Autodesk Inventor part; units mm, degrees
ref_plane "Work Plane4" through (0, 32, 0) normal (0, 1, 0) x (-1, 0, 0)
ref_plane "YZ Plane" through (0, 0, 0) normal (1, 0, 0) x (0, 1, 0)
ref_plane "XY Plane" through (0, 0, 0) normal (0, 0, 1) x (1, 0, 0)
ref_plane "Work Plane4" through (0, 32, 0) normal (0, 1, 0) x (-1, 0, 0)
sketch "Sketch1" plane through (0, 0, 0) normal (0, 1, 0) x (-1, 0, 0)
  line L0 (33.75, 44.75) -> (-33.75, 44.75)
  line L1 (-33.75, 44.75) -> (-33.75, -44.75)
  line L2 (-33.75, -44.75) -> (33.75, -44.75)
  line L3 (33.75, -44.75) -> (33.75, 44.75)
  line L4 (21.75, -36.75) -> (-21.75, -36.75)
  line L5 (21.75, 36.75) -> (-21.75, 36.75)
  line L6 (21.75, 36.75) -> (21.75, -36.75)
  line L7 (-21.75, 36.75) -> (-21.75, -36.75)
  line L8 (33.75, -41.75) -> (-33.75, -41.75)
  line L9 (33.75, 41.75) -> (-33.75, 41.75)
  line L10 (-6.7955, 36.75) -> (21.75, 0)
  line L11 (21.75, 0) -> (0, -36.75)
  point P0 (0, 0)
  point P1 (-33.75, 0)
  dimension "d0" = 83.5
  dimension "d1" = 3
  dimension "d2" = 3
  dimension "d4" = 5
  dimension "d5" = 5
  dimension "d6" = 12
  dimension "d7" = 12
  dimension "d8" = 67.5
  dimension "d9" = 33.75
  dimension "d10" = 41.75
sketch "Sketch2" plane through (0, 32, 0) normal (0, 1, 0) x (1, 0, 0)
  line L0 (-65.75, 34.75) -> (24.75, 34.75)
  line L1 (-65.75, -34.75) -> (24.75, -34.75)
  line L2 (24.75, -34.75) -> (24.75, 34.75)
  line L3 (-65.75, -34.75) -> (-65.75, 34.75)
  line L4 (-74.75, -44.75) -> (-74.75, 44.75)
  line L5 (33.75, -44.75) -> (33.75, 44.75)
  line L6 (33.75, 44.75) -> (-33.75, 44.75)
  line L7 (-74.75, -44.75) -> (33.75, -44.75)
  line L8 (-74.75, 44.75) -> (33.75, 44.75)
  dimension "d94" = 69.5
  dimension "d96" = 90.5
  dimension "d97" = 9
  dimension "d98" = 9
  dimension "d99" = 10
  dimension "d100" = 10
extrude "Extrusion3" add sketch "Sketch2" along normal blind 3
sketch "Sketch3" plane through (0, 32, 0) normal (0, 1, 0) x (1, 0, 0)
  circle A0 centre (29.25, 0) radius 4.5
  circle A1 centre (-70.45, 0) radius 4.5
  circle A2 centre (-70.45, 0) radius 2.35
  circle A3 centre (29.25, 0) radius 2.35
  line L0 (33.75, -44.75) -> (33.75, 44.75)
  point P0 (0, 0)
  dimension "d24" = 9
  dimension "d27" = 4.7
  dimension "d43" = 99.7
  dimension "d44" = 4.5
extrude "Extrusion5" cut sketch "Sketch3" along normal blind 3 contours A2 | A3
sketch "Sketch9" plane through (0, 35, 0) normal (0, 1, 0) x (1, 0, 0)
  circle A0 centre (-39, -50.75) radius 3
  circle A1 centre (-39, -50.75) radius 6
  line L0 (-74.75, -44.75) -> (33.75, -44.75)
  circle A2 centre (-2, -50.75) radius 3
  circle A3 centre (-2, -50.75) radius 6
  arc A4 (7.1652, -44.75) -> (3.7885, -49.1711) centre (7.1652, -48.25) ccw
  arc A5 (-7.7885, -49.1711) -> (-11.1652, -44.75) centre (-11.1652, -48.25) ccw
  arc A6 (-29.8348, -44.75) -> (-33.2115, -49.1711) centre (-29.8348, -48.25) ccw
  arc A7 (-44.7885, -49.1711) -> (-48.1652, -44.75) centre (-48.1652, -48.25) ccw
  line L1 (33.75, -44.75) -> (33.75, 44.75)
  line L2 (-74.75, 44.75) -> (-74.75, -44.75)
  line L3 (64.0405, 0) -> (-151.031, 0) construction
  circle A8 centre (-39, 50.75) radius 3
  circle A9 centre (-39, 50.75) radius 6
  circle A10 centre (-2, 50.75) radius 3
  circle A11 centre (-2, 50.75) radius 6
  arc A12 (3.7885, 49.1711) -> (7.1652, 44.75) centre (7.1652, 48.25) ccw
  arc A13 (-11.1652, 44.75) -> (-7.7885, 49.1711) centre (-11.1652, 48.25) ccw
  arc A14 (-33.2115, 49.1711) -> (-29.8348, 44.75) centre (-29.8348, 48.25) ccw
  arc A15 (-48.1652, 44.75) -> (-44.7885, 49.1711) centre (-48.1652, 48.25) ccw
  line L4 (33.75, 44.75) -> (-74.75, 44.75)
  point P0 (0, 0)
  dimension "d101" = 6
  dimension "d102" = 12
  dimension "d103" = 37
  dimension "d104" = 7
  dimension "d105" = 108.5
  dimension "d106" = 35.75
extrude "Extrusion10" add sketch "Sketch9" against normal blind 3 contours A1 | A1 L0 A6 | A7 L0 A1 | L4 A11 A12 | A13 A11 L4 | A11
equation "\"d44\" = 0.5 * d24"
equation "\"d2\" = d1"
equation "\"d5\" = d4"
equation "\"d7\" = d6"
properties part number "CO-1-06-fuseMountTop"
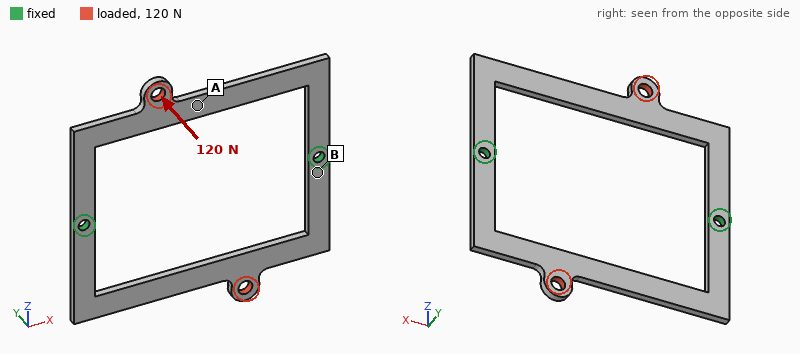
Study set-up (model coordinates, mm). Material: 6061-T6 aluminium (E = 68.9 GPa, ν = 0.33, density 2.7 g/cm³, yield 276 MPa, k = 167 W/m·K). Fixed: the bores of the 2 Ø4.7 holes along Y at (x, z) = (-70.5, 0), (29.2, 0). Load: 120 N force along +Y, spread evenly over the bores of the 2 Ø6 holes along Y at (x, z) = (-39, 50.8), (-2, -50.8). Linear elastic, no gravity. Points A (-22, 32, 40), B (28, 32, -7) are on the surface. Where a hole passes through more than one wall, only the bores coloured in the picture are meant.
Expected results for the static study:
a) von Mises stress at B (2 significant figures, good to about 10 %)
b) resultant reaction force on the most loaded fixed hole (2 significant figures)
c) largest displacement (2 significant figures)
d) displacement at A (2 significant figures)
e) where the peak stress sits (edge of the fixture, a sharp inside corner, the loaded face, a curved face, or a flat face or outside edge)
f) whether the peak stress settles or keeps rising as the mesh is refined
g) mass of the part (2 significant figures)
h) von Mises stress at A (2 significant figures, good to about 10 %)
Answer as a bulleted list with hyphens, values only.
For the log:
- 120 MPa
- 60 N
- 1.5 mm
- 0.91 mm
- edge of the fixture
- keeps rising
- 29 g
- 47 MPa
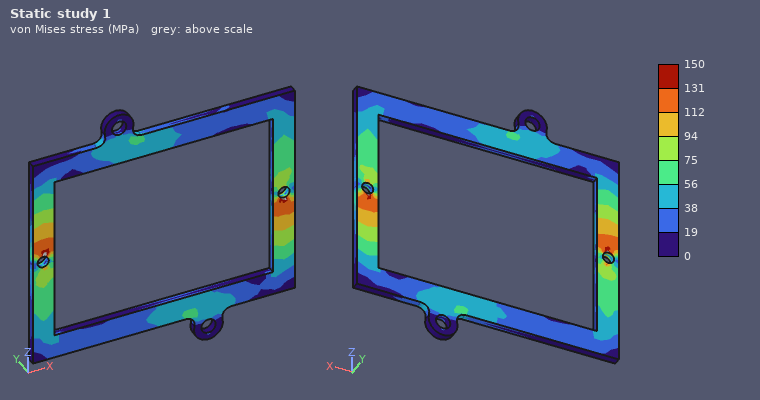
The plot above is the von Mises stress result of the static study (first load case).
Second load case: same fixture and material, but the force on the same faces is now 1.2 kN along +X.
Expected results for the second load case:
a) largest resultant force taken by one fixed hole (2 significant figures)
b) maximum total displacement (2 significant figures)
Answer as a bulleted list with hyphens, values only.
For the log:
- 600 N
- 0.25 mm
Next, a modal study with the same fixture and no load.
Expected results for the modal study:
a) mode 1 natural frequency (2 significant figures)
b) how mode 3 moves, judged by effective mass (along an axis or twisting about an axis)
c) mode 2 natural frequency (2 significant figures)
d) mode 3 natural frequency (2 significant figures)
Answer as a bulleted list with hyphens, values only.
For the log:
- 510 Hz
- twisting about Z
- 510 Hz
- 1200 Hz
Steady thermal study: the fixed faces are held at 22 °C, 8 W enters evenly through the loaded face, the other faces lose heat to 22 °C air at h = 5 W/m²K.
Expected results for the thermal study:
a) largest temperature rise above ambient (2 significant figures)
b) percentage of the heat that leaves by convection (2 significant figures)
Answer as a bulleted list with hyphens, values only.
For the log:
- 37 K
- 9.8 %
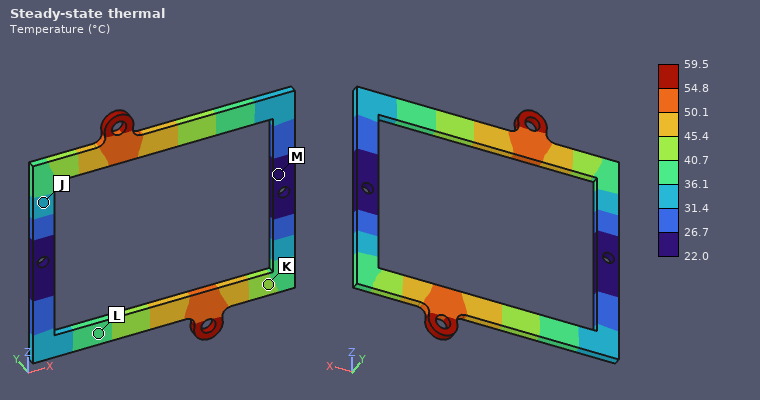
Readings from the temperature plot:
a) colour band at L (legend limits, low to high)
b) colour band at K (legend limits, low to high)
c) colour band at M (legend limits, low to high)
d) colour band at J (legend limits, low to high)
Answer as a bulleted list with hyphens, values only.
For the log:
- 36.1 to 40.7 °C
- 40.7 to 45.4 °C
- 22.0 to 26.7 °C
- 31.4 to 36.1 °C
